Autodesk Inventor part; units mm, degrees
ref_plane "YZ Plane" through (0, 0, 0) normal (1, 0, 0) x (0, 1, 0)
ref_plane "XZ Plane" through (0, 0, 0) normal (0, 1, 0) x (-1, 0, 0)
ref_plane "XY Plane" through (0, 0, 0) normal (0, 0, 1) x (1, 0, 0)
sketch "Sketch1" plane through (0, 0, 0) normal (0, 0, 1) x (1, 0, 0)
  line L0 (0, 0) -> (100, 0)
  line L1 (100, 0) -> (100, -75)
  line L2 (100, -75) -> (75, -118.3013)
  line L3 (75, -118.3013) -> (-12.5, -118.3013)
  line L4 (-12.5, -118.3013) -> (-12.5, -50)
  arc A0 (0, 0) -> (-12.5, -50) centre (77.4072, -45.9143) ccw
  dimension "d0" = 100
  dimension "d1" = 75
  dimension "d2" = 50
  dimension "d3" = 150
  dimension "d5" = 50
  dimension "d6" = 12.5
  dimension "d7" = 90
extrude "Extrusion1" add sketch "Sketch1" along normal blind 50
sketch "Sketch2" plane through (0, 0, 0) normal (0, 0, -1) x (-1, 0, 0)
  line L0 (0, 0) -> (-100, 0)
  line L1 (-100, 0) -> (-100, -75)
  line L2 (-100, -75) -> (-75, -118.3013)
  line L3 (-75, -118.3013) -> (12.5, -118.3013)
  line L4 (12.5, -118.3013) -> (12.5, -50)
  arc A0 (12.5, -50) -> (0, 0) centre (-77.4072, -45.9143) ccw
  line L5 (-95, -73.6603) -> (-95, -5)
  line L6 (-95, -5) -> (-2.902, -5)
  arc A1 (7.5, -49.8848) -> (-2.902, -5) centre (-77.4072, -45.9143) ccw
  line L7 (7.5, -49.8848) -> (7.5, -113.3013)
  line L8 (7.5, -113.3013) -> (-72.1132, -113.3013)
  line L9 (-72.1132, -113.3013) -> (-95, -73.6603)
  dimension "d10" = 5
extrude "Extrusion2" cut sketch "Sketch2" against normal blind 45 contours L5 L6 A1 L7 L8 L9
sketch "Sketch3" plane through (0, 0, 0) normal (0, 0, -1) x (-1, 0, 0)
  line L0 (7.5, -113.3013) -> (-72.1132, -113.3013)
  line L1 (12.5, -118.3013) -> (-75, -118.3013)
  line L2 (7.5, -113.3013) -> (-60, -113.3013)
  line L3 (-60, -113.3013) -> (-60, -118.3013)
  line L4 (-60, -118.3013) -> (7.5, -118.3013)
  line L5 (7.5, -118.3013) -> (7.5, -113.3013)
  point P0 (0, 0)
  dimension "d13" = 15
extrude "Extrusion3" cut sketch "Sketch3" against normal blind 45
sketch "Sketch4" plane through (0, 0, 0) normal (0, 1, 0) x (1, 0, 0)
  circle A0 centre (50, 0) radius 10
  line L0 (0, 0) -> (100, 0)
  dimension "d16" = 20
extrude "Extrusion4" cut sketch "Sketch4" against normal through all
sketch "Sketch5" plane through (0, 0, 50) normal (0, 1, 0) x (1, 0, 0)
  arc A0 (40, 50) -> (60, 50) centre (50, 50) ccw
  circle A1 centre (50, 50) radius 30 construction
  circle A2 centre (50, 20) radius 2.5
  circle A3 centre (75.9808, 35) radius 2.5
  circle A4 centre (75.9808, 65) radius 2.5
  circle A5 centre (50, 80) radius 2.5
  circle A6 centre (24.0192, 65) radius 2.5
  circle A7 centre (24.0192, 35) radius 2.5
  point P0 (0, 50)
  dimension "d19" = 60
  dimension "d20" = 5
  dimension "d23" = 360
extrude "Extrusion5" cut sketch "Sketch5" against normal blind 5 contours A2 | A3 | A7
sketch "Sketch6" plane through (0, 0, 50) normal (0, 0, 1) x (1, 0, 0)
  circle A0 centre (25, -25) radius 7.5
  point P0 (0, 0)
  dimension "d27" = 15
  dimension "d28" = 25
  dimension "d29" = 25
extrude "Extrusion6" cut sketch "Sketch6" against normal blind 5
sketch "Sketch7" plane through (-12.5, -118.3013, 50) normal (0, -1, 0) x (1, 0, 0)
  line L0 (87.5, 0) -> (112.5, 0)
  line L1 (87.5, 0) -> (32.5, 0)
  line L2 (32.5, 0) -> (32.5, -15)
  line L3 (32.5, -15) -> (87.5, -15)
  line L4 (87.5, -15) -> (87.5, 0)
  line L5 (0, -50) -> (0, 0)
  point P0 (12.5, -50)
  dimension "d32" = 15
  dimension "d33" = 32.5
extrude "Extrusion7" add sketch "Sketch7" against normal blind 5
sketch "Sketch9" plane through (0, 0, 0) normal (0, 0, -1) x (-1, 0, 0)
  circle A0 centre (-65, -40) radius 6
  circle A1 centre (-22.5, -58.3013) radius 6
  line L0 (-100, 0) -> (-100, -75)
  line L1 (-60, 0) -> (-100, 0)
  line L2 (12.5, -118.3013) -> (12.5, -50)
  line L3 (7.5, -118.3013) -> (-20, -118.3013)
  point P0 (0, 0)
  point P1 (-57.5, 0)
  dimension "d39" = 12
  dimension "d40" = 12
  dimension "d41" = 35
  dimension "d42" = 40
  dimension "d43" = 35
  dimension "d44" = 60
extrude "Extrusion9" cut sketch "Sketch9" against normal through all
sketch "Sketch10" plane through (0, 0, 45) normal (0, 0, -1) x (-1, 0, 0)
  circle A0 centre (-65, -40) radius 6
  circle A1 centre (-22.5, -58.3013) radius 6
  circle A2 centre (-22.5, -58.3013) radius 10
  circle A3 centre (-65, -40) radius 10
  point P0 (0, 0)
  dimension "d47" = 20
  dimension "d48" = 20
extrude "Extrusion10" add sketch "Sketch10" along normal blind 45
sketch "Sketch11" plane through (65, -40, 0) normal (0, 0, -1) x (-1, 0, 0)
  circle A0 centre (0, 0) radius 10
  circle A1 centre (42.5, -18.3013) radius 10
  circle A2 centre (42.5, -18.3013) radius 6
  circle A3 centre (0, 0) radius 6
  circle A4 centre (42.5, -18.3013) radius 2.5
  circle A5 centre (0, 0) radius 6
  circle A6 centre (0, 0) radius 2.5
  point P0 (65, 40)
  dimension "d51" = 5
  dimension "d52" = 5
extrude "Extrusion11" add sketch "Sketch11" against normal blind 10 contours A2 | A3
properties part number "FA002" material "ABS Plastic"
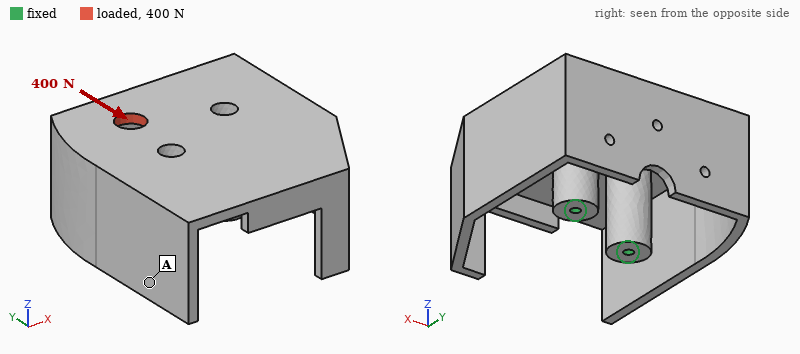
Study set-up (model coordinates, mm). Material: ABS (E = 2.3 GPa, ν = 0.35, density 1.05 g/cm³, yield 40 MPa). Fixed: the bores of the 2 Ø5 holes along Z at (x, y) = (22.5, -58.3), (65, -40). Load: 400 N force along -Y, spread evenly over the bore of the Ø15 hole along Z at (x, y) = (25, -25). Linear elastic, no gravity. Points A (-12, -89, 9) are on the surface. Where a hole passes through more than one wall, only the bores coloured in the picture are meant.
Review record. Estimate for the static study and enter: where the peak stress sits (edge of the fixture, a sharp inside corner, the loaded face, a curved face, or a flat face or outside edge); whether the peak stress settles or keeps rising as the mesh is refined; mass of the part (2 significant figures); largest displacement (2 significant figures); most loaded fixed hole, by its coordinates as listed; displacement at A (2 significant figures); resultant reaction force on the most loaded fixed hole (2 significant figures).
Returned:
edge of the fixture
keeps rising
170 g
1.6 mm
(22.5, -58.3)
0.60 mm
290 N
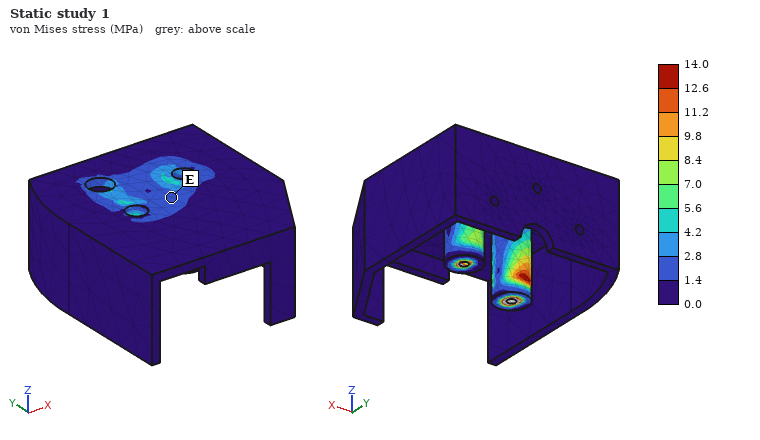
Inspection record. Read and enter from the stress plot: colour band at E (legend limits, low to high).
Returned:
1.4 to 2.8 MPa
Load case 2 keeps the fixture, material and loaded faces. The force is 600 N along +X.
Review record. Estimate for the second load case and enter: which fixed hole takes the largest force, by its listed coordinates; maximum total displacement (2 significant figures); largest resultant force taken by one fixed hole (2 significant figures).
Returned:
(65, -40)
1.9 mm
430 N
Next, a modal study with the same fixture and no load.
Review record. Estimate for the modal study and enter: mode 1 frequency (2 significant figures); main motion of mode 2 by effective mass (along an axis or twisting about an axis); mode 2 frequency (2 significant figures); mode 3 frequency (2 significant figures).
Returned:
160 Hz
twisting about Z
220 Hz
270 Hz
